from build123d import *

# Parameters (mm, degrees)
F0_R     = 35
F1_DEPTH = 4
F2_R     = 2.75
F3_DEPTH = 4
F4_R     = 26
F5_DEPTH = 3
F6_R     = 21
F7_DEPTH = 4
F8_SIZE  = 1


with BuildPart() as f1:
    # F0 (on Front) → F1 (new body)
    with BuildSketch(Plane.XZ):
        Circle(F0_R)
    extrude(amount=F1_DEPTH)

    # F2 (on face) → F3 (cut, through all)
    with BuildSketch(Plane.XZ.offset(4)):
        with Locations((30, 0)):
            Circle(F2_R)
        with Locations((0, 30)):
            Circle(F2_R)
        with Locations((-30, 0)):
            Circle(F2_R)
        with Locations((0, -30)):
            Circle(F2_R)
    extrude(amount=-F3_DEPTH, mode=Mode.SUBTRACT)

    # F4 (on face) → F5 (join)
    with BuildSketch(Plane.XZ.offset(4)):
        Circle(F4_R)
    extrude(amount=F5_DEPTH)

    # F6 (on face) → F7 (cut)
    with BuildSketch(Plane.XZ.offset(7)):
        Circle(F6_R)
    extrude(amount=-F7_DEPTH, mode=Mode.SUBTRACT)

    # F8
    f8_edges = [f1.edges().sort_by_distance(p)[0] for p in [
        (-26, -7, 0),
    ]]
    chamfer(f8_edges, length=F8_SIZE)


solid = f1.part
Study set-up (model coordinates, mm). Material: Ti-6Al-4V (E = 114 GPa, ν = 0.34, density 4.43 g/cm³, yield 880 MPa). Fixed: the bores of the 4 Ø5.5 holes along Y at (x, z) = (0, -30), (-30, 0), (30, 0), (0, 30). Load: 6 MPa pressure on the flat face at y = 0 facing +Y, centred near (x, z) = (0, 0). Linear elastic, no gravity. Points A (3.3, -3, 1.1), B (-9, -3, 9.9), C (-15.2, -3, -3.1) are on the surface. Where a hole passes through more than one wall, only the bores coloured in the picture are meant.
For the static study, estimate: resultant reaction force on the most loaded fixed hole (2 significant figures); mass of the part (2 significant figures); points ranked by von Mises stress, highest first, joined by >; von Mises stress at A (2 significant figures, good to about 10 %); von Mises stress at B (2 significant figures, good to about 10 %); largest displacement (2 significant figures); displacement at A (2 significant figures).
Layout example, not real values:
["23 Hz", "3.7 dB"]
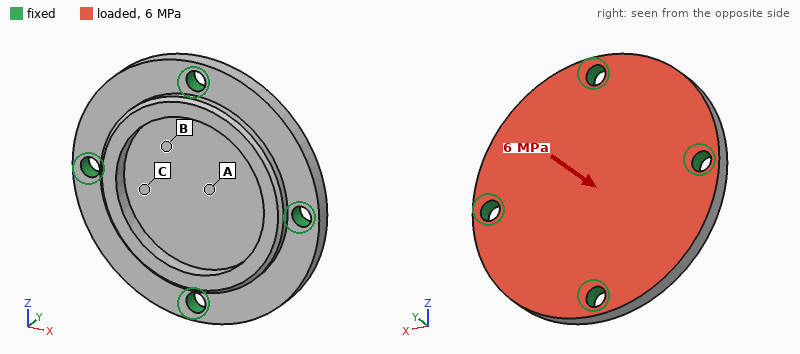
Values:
["5.6 kN", "70 g", "A > B > C", "190 MPa", "110 MPa", "0.18 mm", "0.17 mm"]
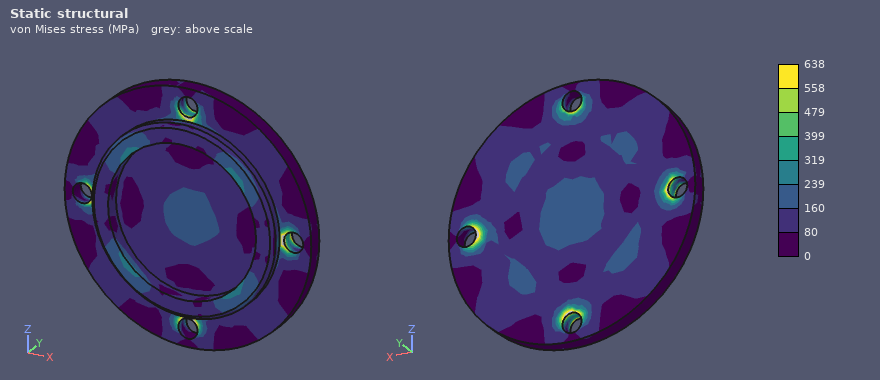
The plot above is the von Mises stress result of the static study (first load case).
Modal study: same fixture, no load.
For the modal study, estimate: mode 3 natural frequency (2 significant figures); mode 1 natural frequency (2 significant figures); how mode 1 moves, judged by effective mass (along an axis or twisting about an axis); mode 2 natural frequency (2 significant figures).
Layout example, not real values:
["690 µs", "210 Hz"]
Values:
["12 kHz", "9700 Hz", "along Y", "11 kHz"]
